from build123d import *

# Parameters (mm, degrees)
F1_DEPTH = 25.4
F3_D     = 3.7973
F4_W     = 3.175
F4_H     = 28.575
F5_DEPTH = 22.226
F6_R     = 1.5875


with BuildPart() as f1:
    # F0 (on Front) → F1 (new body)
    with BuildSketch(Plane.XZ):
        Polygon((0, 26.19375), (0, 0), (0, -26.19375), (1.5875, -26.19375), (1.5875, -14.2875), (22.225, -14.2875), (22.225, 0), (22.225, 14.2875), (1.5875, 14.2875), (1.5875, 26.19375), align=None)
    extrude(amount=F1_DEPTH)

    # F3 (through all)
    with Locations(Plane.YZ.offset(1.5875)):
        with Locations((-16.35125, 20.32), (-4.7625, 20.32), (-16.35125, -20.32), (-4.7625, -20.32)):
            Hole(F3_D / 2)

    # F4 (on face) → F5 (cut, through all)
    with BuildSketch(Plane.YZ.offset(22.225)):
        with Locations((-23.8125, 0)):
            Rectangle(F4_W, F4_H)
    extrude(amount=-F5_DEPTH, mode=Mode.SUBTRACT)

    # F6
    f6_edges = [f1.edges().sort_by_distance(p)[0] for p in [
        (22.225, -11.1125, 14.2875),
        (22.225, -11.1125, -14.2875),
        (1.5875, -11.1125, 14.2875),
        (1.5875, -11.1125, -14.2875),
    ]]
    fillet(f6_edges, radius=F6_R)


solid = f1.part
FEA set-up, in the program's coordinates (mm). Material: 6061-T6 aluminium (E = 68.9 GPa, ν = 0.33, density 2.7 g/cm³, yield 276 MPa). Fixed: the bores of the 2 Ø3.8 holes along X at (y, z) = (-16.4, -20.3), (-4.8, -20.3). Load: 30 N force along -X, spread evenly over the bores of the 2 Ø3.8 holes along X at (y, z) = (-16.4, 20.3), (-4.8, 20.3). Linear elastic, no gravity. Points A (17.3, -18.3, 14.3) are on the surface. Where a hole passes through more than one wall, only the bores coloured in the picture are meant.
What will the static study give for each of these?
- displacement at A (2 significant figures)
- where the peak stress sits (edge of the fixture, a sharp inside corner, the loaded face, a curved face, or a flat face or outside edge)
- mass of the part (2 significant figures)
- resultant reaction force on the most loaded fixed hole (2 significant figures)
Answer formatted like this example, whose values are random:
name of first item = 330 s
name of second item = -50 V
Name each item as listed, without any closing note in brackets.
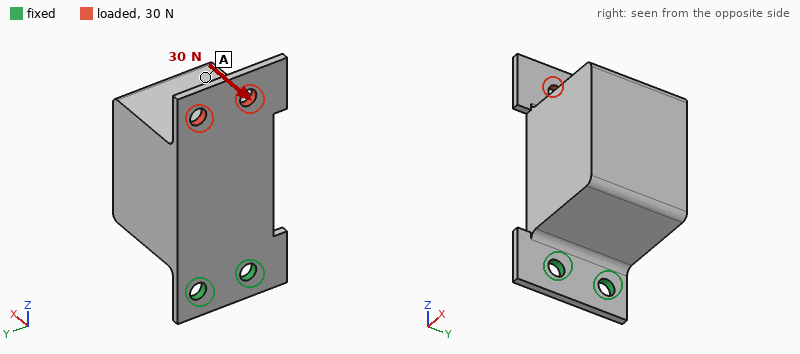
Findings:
displacement at A = 0.34 mm
where the peak stress sits = a flat face or outside edge
mass of the part = 41 g
resultant reaction force on the most loaded fixed hole = 15 N
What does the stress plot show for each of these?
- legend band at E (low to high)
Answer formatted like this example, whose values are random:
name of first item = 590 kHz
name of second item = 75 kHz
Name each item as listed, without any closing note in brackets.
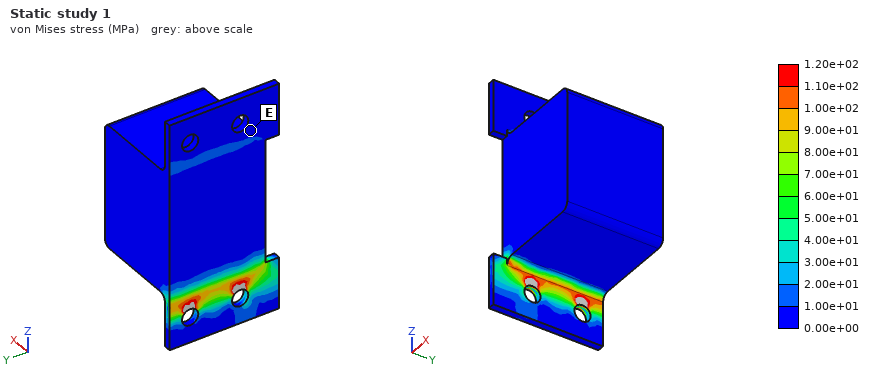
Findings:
legend band at E = 0.00e+00 to 1.00e+01 MPa
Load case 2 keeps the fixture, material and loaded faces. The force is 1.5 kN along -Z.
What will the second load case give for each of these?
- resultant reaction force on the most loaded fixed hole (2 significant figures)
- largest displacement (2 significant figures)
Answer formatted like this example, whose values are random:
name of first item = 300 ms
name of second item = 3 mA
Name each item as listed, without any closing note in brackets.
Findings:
resultant reaction force on the most loaded fixed hole = 760 N
largest displacement = 71 µm
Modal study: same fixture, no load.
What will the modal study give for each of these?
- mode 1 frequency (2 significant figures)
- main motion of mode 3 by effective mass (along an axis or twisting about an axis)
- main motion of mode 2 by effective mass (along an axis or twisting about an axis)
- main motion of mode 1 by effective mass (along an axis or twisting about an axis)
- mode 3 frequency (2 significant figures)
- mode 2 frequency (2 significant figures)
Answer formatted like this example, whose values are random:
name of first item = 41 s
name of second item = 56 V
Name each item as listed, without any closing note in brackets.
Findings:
mode 1 frequency = 380 Hz
main motion of mode 3 by effective mass = along Y
main motion of mode 2 by effective mass = along Y
main motion of mode 1 by effective mass = along X
mode 3 frequency = 4400 Hz
mode 2 frequency = 2100 Hz
